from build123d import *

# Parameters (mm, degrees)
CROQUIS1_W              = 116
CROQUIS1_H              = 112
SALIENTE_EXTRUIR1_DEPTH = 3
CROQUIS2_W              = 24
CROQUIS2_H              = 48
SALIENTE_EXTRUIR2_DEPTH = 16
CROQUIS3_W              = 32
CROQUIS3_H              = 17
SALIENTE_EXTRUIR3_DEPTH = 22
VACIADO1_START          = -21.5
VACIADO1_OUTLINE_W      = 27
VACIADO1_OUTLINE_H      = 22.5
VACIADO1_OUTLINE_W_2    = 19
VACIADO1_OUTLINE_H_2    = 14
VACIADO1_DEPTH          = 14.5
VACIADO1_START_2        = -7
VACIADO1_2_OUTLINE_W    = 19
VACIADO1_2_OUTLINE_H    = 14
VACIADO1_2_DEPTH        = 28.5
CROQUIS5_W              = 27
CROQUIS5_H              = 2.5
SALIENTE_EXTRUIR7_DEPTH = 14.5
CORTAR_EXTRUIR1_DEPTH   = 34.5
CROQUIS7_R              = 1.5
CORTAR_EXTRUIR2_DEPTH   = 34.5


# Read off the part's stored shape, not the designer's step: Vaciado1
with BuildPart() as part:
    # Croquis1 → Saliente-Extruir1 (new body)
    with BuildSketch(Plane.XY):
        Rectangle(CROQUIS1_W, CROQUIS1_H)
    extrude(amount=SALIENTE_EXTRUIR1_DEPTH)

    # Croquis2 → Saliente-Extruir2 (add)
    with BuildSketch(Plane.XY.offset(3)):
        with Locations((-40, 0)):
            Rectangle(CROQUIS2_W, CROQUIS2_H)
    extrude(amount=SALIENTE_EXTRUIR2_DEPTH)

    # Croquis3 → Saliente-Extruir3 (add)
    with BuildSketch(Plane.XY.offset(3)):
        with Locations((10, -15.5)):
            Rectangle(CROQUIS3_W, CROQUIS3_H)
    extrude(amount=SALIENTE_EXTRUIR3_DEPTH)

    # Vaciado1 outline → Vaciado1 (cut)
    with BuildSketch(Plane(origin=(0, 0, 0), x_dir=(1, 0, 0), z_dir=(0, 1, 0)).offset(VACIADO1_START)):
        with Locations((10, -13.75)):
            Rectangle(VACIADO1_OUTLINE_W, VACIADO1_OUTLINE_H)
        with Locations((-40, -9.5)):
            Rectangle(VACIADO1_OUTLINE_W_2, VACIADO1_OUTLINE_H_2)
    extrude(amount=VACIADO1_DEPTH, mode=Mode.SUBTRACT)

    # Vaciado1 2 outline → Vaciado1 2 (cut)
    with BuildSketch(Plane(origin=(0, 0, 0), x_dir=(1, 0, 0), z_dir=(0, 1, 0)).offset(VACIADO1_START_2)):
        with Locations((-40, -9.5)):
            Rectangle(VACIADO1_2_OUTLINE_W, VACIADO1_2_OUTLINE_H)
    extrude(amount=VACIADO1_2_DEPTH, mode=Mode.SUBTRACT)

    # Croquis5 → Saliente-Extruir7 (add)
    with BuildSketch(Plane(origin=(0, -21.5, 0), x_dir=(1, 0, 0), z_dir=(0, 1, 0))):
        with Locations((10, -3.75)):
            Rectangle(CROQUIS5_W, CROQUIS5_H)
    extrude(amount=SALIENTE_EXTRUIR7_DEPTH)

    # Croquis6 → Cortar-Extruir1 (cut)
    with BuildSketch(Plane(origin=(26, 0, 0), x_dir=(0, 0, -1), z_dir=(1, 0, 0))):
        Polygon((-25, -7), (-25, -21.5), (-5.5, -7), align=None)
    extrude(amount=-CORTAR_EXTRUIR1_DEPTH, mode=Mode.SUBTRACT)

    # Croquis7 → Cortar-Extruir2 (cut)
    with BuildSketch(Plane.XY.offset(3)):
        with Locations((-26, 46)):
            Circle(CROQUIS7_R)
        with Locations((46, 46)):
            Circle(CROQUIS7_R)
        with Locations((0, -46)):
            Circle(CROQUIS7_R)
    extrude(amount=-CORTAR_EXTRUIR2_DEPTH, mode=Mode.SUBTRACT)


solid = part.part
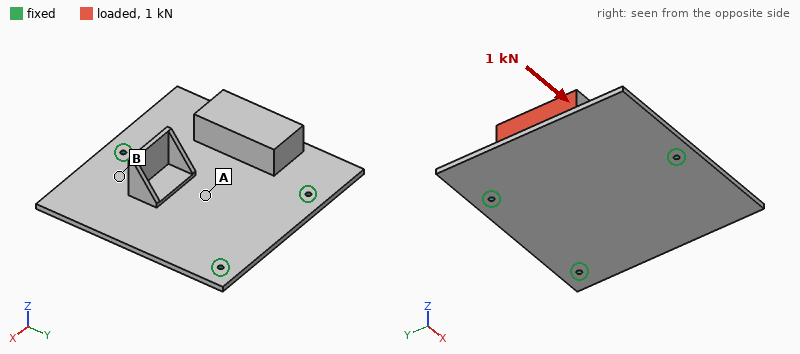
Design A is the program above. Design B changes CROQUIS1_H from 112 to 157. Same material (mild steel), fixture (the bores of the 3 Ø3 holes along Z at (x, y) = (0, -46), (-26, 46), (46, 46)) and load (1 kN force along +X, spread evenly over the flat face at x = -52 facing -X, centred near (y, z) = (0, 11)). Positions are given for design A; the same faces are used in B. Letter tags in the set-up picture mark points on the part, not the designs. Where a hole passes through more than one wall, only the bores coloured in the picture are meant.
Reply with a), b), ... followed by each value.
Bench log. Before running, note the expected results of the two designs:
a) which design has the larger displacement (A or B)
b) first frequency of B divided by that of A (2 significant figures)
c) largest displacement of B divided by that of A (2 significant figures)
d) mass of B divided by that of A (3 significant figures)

a) A
b) 0.90
c) 0.86
d) 1.32
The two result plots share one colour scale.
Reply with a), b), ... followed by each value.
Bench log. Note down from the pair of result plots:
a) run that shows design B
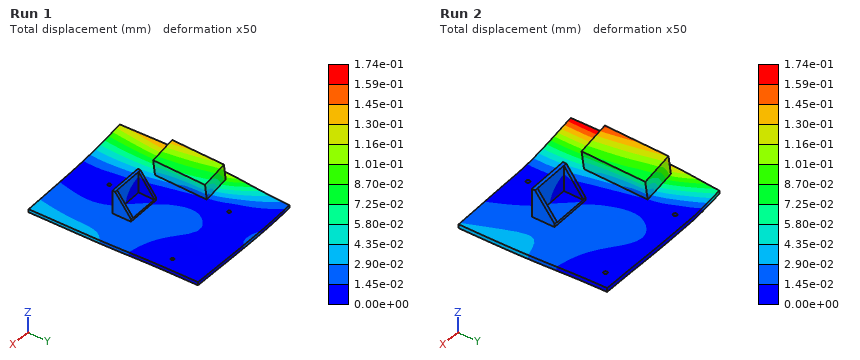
a) Run 1
